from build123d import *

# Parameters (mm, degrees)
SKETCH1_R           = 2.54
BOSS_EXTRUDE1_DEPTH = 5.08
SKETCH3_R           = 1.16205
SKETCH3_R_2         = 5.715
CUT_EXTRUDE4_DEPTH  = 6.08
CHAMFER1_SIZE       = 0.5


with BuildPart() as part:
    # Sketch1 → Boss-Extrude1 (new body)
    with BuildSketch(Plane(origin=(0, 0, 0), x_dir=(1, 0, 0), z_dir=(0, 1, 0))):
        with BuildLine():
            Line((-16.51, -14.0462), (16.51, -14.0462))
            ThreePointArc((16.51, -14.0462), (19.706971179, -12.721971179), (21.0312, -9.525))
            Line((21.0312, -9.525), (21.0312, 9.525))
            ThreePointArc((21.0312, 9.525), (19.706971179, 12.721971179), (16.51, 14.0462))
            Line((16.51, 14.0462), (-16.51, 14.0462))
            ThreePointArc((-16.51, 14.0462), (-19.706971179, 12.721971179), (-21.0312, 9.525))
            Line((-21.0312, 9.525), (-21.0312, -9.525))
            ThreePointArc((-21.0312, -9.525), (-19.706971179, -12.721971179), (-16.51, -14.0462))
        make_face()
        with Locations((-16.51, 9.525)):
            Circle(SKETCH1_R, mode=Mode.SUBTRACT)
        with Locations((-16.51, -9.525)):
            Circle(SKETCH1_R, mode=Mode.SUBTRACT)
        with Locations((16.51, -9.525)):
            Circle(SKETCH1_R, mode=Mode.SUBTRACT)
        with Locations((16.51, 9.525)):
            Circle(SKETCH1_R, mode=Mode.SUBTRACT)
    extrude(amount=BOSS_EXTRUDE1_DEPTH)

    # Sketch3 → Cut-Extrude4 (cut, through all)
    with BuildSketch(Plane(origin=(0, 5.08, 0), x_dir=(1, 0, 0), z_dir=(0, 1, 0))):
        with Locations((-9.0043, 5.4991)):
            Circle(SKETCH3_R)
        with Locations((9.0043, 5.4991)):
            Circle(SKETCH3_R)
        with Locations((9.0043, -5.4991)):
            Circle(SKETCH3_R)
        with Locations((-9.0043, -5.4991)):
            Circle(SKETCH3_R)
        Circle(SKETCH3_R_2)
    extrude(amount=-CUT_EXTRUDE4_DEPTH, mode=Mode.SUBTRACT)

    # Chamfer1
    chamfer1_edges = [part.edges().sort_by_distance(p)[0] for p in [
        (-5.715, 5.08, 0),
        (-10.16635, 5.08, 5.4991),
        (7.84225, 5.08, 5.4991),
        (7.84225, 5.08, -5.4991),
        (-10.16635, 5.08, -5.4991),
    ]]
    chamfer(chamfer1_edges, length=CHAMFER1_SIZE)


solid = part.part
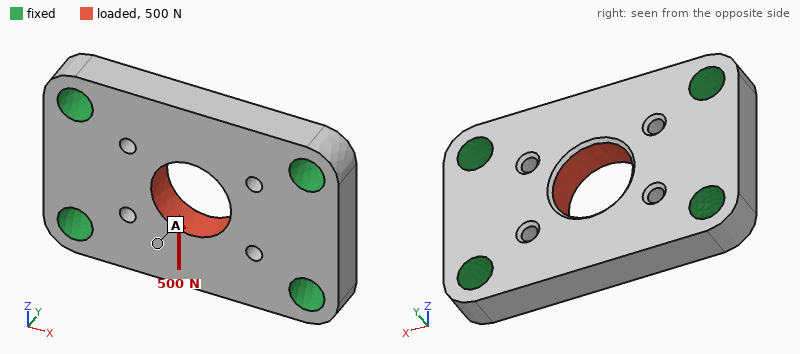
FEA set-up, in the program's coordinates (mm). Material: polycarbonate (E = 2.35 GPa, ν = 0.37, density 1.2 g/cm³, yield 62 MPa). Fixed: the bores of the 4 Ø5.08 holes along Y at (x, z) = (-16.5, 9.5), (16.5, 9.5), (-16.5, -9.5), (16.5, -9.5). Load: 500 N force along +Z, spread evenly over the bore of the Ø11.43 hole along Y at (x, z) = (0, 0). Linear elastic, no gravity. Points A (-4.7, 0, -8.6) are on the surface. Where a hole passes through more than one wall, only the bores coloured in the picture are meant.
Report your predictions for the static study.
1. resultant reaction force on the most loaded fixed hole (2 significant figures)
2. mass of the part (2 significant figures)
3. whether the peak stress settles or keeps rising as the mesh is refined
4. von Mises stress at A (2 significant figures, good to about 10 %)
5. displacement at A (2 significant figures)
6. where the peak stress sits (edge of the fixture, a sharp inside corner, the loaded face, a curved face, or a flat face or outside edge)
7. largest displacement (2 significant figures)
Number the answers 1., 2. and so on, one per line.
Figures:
1. 150 N
2. 5.9 g
3. keeps rising
4. 2.9 MPa
5. 31 µm
6. a sharp inside corner
7. 41 µm
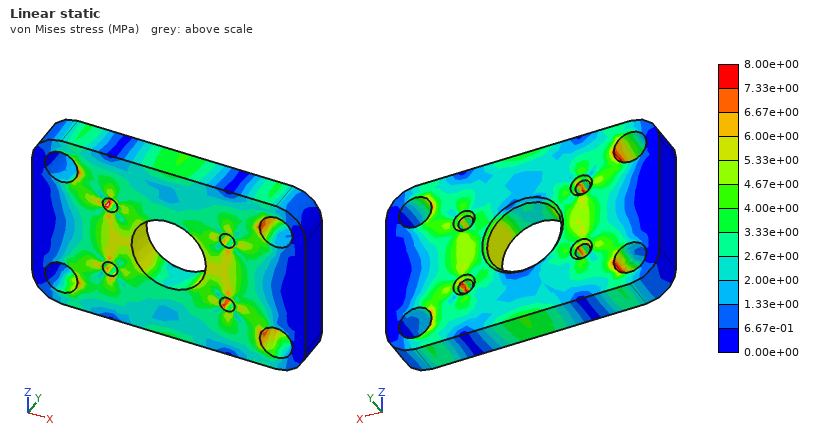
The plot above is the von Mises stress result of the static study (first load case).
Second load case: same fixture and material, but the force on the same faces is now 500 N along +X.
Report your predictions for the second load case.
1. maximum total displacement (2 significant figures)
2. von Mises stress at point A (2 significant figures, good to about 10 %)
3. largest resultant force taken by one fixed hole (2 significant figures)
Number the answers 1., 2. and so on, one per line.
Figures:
1. 17 µm
2. 1.9 MPa
3. 130 N
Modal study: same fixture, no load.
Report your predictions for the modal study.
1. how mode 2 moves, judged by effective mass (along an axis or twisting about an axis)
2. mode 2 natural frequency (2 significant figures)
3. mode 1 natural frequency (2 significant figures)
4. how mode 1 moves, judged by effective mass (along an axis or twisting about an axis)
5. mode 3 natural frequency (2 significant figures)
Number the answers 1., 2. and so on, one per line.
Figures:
1. twisting about X
2. 8000 Hz
3. 6900 Hz
4. along Y
5. 12 kHz
